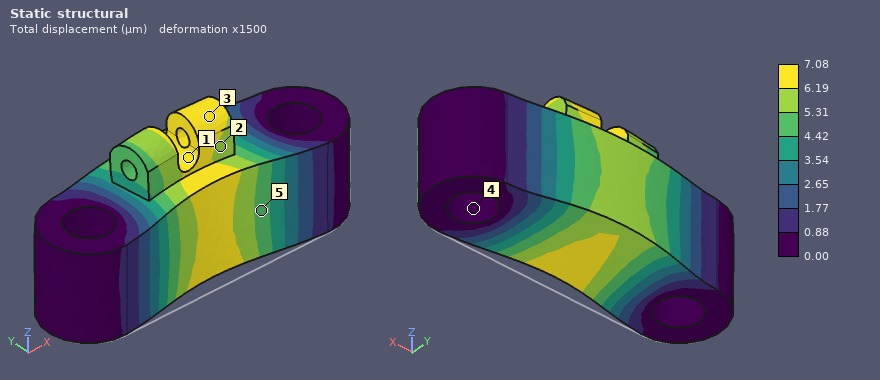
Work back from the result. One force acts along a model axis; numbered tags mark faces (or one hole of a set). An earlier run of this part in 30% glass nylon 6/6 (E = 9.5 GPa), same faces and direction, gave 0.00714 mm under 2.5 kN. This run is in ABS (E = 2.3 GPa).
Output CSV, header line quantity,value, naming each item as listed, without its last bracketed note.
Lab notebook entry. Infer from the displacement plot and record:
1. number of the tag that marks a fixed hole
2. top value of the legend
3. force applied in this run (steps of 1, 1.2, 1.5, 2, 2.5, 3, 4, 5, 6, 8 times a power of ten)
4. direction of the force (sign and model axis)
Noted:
quantity,value
number of the tag that marks a fixed hole,4
top value of the legend,7.08 µm
force applied in this run,600 N
direction of the force,+Y
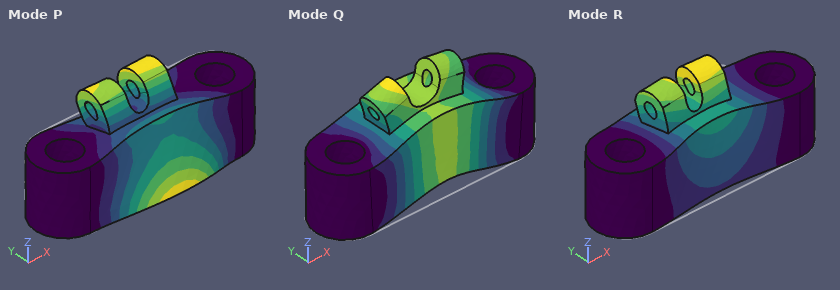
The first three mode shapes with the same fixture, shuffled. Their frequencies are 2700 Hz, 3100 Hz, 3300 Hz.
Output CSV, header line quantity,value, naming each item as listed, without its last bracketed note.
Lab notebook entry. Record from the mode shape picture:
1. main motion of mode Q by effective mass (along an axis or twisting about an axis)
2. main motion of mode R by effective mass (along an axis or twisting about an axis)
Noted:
quantity,value
main motion of mode Q by effective mass,along Z
main motion of mode R by effective mass,along Y
